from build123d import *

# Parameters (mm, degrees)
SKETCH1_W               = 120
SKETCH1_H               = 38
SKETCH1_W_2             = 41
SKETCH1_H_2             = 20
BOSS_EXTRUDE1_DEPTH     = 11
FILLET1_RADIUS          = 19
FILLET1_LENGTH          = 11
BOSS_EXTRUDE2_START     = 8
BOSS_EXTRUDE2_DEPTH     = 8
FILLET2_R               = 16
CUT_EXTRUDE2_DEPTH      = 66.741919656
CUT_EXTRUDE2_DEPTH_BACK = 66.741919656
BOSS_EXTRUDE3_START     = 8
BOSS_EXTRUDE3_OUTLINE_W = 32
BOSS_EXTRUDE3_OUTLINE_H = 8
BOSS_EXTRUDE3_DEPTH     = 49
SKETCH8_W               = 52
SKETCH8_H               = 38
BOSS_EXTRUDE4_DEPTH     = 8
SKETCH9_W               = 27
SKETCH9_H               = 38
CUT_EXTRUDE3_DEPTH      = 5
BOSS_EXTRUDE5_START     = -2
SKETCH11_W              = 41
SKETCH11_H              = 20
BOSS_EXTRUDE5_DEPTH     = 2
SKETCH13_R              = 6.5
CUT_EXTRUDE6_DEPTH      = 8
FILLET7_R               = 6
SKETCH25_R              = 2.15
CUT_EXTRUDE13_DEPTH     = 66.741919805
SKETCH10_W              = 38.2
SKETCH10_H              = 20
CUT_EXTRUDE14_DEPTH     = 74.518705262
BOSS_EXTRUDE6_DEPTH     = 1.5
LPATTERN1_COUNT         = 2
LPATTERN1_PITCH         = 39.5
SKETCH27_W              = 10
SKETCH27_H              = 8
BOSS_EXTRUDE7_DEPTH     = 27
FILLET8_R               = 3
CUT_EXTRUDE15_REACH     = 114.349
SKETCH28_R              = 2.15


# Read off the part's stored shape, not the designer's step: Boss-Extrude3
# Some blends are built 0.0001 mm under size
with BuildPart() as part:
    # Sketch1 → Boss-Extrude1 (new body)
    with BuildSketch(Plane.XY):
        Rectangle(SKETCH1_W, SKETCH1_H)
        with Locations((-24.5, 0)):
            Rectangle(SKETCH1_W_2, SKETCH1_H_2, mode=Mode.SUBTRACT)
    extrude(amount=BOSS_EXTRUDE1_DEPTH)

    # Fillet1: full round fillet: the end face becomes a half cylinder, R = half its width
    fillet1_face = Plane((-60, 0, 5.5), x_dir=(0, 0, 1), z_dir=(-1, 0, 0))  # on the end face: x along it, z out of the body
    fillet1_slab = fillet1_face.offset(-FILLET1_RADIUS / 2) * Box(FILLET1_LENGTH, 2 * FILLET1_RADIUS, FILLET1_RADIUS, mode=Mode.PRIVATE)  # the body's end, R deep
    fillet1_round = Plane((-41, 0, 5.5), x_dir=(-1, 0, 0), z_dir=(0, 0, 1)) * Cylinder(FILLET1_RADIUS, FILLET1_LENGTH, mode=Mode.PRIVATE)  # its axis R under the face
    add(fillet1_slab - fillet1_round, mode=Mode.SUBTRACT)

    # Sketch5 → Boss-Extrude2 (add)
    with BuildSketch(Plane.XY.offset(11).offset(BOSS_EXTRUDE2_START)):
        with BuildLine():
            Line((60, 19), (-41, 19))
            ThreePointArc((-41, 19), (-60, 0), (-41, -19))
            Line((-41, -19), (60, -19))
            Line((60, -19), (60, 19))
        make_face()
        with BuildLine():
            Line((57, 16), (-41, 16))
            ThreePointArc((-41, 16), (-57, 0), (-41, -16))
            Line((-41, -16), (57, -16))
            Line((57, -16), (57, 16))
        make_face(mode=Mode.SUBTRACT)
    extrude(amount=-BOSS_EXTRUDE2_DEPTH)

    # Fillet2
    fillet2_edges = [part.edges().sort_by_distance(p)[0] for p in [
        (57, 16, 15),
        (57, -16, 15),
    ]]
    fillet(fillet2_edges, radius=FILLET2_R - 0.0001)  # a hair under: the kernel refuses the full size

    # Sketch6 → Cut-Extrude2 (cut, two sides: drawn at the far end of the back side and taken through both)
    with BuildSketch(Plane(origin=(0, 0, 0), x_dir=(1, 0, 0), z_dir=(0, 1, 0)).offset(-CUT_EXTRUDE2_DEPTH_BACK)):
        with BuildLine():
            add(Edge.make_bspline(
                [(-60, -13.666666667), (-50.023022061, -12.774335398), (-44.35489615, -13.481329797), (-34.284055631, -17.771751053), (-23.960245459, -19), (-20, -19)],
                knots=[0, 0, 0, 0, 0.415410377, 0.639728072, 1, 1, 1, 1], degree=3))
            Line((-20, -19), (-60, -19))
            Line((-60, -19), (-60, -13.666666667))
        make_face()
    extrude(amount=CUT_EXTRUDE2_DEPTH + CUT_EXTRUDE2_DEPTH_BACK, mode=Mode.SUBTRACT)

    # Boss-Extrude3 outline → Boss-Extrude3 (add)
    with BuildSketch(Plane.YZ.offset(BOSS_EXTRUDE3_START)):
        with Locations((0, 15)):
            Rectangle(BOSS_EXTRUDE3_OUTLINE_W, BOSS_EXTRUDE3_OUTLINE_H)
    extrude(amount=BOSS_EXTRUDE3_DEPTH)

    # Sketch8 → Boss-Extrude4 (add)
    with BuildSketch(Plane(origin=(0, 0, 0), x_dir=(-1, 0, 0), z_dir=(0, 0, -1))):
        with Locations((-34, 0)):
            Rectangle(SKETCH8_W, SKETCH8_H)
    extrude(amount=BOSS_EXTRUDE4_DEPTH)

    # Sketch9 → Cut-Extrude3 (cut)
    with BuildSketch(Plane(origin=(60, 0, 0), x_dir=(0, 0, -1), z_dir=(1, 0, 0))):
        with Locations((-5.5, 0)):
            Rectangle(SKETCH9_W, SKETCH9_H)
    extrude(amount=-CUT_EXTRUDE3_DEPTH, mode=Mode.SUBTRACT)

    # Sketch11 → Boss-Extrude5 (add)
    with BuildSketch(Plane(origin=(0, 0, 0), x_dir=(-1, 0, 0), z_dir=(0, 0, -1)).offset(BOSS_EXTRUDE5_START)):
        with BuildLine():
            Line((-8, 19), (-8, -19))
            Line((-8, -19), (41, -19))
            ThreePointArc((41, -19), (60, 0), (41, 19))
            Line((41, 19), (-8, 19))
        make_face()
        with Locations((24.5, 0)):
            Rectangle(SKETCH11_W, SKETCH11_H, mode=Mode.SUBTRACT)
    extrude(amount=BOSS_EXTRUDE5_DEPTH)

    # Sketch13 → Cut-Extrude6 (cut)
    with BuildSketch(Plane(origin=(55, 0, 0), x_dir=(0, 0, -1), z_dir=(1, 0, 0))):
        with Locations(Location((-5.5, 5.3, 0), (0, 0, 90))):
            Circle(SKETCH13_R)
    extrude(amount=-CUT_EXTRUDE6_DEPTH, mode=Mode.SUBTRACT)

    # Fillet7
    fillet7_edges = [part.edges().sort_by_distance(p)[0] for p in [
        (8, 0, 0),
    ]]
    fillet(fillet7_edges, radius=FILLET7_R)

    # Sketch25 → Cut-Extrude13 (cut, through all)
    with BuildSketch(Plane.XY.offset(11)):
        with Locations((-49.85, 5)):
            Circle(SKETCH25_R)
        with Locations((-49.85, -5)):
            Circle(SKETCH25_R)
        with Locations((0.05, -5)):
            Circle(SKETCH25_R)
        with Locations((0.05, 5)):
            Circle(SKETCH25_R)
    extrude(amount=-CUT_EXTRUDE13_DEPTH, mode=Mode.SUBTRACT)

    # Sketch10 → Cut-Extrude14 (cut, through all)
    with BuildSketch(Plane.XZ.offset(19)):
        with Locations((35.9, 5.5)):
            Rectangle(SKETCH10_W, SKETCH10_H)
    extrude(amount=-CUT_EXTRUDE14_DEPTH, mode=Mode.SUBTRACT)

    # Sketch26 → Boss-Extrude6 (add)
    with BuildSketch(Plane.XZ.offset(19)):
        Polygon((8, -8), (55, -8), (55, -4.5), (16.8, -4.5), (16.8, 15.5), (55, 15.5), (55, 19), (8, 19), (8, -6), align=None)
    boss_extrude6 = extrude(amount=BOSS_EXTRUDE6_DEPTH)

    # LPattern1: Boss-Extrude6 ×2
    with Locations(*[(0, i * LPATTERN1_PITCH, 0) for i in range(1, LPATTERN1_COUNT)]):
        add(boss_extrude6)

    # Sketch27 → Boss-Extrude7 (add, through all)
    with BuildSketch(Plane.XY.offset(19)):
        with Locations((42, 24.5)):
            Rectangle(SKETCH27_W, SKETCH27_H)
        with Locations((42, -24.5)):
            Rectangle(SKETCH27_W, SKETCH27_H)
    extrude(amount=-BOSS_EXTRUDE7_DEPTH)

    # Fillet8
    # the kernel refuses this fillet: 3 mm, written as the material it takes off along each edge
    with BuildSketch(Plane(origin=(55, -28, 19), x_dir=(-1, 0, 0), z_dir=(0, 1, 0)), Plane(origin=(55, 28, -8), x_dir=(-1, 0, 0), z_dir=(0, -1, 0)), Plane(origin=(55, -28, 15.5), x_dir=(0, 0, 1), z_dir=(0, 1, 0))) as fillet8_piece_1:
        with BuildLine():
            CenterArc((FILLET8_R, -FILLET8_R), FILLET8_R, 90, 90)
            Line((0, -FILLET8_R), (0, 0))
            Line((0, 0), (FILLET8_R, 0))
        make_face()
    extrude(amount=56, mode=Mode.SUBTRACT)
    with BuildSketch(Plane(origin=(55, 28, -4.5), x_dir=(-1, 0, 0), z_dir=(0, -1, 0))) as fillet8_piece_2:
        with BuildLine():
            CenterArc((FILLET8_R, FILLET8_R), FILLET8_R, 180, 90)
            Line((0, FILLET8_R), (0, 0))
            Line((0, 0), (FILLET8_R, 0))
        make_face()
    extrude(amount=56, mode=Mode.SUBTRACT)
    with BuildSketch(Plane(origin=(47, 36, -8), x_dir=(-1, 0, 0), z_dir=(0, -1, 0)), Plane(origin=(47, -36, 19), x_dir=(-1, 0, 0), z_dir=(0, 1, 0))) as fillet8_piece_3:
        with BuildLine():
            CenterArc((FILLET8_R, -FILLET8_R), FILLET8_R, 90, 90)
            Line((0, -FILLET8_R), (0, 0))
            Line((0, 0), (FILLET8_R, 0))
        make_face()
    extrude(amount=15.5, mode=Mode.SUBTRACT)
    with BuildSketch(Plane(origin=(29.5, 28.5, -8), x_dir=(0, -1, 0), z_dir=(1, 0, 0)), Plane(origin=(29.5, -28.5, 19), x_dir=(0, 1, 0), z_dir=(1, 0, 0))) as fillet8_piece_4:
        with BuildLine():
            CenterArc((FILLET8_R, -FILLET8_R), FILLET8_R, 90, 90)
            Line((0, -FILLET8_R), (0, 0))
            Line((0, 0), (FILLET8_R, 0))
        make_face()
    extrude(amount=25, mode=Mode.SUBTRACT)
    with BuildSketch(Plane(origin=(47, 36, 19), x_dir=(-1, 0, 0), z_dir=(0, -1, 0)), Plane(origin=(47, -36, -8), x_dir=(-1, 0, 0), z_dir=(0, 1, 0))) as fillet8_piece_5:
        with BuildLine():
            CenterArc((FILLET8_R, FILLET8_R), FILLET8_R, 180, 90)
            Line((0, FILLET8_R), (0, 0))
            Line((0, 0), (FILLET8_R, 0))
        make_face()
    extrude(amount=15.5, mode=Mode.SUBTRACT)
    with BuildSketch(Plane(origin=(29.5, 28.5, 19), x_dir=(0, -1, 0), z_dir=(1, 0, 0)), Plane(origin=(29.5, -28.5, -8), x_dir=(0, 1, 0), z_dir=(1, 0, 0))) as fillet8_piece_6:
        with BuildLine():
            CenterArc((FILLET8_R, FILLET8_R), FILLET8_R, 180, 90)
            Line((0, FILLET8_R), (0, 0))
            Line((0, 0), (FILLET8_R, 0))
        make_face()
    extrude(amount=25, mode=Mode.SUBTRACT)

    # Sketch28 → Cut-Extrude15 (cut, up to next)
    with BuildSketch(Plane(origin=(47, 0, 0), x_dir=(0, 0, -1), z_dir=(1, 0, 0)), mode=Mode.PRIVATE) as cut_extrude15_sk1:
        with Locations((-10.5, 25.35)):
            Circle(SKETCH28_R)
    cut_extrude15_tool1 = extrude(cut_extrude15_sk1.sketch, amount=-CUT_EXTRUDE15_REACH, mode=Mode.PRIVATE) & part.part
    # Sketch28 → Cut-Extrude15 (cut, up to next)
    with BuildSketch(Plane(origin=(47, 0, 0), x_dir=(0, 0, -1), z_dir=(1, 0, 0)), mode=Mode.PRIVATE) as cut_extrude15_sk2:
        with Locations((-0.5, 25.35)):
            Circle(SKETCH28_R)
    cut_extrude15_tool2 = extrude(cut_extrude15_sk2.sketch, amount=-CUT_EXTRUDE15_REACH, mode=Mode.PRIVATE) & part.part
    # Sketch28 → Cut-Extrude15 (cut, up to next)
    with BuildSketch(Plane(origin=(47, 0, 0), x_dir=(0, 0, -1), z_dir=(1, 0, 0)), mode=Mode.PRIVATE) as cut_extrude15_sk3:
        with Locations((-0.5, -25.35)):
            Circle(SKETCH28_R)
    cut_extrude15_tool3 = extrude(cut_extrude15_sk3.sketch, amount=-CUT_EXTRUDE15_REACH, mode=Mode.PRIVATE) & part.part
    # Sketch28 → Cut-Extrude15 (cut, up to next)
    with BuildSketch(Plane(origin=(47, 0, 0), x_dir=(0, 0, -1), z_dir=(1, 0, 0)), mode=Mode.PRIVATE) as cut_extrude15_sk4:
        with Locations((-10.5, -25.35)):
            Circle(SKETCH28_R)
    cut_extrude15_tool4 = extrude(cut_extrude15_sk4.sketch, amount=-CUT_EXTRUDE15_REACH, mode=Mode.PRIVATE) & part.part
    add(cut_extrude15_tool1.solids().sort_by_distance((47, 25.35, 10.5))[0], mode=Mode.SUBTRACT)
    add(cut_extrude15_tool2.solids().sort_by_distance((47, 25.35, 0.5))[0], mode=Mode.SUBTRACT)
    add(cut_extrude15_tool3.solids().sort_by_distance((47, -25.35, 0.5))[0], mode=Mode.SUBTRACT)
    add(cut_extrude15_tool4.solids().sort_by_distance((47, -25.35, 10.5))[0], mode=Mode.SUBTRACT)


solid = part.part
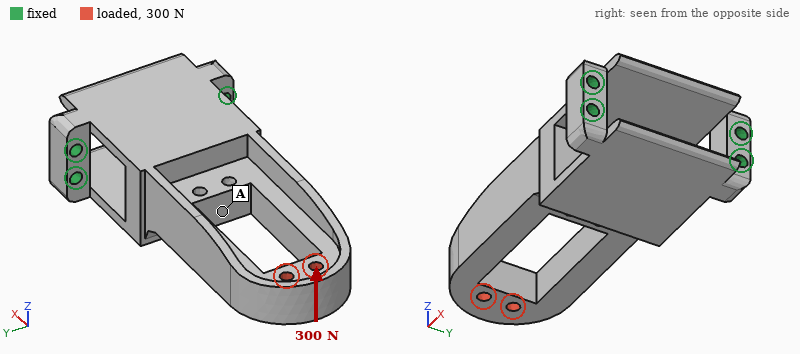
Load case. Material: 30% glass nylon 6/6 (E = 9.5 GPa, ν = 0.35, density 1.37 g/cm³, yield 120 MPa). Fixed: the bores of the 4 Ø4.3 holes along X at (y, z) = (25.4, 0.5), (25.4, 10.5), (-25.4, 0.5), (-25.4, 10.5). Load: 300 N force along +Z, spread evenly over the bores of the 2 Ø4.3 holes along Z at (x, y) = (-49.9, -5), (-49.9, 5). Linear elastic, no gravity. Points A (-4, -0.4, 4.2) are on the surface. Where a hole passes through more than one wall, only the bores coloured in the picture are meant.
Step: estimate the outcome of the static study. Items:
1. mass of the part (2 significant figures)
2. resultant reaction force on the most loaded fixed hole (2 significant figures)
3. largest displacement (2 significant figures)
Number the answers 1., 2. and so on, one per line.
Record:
1. 60 g
2. 540 N
3. 1.3 mm
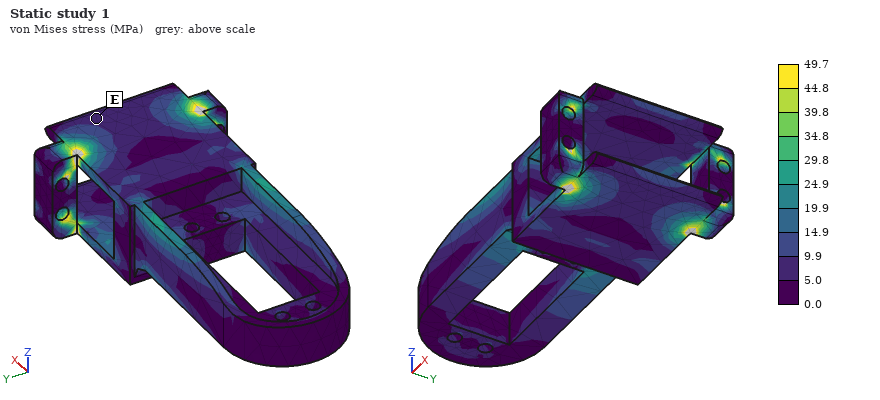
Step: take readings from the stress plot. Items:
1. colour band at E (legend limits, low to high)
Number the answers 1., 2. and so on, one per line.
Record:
1. 5.0 to 9.9 MPa
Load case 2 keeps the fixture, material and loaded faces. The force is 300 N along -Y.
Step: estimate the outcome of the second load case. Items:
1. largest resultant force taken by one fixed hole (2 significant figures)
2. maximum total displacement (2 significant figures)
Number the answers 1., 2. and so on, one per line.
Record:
1. 320 N
2. 0.62 mm
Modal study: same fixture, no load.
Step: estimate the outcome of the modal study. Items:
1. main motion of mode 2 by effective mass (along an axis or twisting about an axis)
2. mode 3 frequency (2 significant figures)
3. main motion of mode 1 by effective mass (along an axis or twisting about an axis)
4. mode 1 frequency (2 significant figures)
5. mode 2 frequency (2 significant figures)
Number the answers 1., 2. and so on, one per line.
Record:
1. along Y
2. 1600 Hz
3. along Z
4. 610 Hz
5. 1000 Hz
